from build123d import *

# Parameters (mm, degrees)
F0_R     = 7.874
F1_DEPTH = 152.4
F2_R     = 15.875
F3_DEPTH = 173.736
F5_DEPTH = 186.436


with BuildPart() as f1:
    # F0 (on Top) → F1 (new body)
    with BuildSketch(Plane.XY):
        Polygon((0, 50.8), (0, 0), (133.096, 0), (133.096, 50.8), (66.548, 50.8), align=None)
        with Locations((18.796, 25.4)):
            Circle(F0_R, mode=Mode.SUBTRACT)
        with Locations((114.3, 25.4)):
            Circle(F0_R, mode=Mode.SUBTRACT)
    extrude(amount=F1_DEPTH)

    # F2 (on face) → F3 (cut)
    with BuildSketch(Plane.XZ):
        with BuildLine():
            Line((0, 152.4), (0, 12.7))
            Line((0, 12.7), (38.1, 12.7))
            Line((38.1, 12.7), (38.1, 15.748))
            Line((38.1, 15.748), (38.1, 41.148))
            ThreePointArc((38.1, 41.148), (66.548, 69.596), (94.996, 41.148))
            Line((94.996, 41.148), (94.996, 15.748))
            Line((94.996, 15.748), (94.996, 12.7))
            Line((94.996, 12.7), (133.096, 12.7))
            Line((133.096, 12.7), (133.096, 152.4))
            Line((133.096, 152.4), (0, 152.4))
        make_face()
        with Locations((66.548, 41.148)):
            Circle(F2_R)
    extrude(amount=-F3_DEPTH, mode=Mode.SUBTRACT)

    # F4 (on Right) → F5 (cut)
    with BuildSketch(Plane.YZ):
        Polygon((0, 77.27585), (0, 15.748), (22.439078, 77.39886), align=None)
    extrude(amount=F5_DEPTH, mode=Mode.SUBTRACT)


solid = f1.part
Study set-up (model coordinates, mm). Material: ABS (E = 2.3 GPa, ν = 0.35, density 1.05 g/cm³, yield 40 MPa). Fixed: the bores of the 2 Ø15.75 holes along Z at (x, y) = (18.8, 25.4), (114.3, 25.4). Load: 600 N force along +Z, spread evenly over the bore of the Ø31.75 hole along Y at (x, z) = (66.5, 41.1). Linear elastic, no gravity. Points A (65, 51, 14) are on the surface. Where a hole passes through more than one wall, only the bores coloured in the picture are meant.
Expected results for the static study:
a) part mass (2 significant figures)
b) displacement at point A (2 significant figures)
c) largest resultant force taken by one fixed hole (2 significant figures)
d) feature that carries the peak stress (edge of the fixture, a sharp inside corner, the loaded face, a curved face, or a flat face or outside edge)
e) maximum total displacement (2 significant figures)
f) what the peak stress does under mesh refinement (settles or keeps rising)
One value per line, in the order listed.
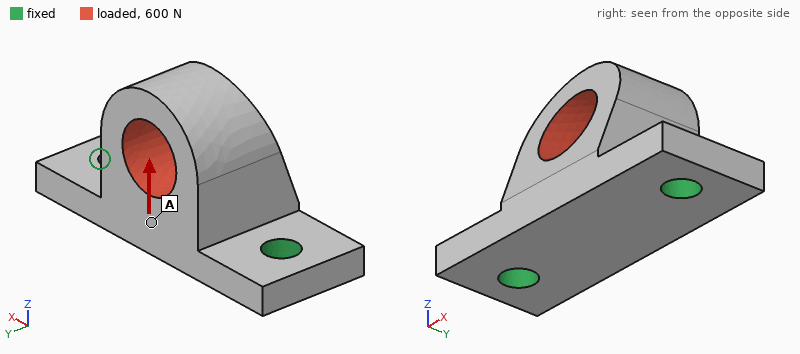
180 g
54 µm
330 N
edge of the fixture
74 µm
keeps rising
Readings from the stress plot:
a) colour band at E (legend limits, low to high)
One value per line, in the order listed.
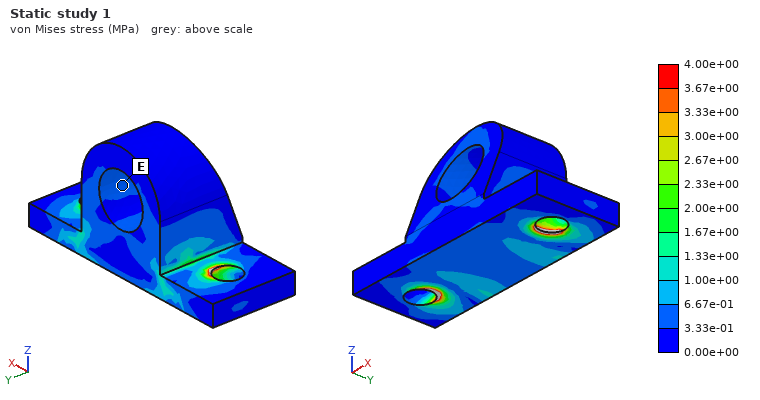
3.33e-01 to 6.67e-01 MPa
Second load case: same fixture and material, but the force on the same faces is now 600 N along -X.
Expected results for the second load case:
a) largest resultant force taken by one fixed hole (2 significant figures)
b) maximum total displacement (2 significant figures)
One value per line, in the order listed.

410 N
90 µm
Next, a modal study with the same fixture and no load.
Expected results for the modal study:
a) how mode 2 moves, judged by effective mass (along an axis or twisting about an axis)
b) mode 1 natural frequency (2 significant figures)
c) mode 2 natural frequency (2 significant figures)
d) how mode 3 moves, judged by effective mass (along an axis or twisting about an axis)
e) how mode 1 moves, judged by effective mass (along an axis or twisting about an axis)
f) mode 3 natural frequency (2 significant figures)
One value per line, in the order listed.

along X
800 Hz
1700 Hz
along Z
along Y
1800 Hz
